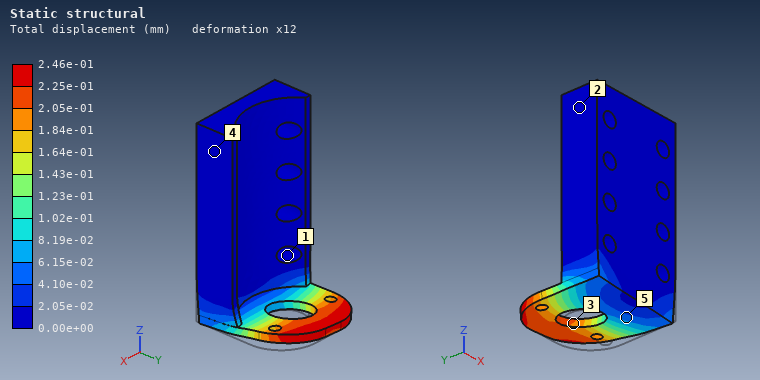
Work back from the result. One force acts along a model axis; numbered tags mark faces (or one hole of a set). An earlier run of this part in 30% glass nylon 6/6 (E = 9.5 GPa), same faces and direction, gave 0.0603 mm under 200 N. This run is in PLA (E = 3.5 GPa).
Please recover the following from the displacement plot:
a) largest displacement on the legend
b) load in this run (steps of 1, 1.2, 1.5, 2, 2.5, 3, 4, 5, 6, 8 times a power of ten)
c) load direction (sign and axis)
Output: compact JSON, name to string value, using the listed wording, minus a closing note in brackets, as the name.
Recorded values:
{"largest displacement on the legend": "2.46e-01 mm", "load in this run": "300 N", "load direction": "-X"}
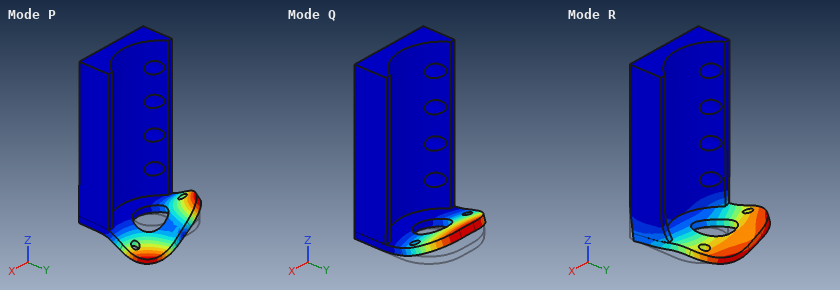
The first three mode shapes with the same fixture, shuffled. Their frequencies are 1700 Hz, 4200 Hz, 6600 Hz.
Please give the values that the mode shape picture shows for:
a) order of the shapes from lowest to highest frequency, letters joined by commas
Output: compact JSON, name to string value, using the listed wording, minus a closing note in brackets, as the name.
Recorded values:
{"order of the shapes from lowest to highest frequency, letters joined by commas": "Q, P, R"}
